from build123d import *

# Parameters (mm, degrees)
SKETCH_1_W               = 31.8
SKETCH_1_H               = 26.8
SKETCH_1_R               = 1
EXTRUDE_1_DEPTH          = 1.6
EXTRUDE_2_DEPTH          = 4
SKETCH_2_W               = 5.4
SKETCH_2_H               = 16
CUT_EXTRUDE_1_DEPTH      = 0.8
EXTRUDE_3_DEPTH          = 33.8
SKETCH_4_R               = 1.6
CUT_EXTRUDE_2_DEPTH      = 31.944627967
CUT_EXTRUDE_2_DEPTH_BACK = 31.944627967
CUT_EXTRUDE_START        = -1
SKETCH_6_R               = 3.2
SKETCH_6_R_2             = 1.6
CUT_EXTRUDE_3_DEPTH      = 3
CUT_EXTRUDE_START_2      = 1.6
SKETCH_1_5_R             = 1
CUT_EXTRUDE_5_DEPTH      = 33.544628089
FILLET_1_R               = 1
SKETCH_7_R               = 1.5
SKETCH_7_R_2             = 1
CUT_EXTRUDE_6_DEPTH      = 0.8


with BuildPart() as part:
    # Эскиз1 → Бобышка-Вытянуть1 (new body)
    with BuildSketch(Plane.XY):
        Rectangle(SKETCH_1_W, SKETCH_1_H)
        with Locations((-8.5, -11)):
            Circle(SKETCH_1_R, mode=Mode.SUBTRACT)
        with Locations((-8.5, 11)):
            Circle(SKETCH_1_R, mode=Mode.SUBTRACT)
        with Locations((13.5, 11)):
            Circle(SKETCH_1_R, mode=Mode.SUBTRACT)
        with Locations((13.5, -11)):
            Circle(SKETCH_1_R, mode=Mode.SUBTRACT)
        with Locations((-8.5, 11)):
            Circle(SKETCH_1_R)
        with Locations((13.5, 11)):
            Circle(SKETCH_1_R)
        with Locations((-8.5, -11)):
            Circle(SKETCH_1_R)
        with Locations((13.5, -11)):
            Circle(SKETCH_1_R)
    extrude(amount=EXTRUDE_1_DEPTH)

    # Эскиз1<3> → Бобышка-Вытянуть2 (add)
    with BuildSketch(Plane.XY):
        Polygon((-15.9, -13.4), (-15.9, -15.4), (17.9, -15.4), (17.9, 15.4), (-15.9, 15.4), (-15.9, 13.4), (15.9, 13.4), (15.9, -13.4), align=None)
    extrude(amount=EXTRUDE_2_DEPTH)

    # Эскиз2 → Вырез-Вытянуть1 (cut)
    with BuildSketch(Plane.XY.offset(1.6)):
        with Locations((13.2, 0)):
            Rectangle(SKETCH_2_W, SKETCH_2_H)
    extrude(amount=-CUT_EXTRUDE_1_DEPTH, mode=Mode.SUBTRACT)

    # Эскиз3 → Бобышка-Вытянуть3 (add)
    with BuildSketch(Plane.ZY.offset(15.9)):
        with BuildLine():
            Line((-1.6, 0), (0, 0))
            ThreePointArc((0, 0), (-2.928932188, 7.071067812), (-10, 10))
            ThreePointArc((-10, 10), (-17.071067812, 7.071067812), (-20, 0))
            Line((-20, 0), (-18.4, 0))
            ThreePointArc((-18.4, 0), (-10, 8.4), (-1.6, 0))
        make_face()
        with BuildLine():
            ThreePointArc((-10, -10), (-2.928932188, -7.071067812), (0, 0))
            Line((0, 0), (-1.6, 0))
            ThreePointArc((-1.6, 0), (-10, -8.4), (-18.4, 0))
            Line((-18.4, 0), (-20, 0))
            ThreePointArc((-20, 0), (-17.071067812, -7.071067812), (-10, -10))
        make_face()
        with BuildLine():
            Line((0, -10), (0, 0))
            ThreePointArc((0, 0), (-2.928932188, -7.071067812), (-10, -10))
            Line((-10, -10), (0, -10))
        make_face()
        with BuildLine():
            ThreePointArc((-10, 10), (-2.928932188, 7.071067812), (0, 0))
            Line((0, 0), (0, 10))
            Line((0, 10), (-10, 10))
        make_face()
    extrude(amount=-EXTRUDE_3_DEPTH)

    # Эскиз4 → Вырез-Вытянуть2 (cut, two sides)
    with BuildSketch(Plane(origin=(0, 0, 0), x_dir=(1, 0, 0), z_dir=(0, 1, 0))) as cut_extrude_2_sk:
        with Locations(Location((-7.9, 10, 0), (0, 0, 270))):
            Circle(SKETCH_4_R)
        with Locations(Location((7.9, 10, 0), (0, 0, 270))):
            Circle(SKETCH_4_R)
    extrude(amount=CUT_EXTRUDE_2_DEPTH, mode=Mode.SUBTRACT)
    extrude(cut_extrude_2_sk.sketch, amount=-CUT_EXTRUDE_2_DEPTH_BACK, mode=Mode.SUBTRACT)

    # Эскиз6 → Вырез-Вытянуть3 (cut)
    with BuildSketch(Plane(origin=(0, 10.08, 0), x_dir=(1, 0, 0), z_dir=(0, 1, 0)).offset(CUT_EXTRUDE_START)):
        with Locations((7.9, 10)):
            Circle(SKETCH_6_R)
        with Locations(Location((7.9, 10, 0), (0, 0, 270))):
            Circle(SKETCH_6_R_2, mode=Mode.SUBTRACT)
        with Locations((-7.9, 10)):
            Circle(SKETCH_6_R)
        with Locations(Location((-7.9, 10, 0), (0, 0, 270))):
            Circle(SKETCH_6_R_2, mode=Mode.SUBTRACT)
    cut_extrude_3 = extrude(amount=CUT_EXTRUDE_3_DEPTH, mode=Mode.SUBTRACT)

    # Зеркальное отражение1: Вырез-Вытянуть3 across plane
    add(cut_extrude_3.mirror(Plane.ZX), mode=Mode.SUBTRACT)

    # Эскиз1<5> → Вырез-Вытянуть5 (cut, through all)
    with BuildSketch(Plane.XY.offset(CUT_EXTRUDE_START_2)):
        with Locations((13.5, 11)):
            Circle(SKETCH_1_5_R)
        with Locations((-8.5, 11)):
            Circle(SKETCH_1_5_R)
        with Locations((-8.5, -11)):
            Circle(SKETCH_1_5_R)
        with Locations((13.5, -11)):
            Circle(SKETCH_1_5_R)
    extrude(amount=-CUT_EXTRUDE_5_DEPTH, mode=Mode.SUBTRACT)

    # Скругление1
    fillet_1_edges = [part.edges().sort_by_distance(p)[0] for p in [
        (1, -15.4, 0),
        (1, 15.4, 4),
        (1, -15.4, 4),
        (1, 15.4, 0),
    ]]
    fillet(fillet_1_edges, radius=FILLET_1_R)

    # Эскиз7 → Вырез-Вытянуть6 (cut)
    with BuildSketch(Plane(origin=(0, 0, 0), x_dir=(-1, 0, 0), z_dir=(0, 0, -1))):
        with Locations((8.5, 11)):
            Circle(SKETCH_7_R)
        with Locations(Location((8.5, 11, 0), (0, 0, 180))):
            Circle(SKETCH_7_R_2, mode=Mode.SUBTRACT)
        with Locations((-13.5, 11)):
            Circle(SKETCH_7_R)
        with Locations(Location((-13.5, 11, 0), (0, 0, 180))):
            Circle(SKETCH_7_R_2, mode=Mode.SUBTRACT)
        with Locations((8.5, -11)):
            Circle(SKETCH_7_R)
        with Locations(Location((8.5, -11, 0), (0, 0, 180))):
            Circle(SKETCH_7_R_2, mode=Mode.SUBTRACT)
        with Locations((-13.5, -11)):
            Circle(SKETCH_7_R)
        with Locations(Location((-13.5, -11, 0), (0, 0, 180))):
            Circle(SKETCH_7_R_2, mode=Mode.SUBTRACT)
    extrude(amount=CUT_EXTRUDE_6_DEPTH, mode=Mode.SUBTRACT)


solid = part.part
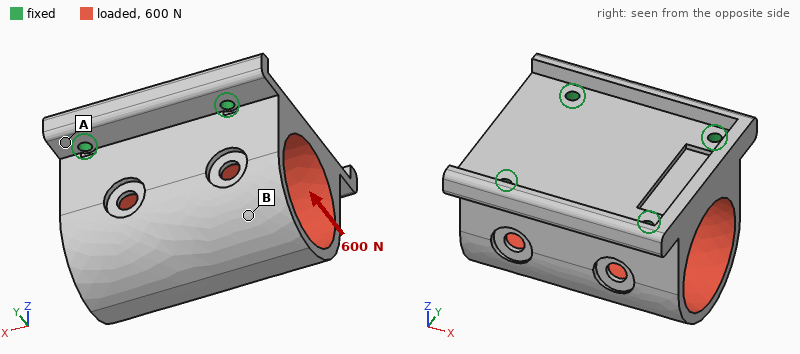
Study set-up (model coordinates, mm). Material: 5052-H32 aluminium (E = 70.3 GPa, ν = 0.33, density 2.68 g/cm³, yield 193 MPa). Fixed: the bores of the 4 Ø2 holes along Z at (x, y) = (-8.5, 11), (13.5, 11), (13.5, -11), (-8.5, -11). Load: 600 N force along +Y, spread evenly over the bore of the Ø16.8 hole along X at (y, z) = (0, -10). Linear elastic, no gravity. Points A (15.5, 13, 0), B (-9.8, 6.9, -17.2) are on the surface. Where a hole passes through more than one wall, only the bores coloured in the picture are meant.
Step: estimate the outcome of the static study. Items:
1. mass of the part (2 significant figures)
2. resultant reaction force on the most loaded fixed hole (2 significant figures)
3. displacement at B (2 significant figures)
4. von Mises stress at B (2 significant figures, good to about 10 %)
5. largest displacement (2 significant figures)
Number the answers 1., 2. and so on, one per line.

1. 17 g
2. 230 N
3. 27 µm
4. 20 MPa
5. 28 µm
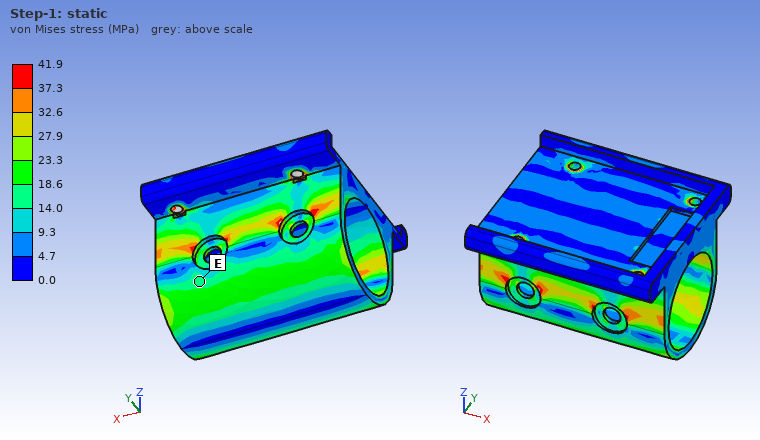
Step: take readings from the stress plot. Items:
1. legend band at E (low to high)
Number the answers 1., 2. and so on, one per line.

1. 14.0 to 18.6 MPa
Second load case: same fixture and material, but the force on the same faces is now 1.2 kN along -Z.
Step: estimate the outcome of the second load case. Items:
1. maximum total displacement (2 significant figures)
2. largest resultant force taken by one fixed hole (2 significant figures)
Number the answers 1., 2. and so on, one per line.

1. 10 µm
2. 370 N
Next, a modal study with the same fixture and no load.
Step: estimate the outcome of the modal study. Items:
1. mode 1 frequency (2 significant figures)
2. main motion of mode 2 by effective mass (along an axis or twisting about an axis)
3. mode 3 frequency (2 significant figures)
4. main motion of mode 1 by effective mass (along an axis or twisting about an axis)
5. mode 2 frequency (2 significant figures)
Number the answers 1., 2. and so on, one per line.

1. 8900 Hz
2. along X
3. 17 kHz
4. along Y
5. 15 kHz
